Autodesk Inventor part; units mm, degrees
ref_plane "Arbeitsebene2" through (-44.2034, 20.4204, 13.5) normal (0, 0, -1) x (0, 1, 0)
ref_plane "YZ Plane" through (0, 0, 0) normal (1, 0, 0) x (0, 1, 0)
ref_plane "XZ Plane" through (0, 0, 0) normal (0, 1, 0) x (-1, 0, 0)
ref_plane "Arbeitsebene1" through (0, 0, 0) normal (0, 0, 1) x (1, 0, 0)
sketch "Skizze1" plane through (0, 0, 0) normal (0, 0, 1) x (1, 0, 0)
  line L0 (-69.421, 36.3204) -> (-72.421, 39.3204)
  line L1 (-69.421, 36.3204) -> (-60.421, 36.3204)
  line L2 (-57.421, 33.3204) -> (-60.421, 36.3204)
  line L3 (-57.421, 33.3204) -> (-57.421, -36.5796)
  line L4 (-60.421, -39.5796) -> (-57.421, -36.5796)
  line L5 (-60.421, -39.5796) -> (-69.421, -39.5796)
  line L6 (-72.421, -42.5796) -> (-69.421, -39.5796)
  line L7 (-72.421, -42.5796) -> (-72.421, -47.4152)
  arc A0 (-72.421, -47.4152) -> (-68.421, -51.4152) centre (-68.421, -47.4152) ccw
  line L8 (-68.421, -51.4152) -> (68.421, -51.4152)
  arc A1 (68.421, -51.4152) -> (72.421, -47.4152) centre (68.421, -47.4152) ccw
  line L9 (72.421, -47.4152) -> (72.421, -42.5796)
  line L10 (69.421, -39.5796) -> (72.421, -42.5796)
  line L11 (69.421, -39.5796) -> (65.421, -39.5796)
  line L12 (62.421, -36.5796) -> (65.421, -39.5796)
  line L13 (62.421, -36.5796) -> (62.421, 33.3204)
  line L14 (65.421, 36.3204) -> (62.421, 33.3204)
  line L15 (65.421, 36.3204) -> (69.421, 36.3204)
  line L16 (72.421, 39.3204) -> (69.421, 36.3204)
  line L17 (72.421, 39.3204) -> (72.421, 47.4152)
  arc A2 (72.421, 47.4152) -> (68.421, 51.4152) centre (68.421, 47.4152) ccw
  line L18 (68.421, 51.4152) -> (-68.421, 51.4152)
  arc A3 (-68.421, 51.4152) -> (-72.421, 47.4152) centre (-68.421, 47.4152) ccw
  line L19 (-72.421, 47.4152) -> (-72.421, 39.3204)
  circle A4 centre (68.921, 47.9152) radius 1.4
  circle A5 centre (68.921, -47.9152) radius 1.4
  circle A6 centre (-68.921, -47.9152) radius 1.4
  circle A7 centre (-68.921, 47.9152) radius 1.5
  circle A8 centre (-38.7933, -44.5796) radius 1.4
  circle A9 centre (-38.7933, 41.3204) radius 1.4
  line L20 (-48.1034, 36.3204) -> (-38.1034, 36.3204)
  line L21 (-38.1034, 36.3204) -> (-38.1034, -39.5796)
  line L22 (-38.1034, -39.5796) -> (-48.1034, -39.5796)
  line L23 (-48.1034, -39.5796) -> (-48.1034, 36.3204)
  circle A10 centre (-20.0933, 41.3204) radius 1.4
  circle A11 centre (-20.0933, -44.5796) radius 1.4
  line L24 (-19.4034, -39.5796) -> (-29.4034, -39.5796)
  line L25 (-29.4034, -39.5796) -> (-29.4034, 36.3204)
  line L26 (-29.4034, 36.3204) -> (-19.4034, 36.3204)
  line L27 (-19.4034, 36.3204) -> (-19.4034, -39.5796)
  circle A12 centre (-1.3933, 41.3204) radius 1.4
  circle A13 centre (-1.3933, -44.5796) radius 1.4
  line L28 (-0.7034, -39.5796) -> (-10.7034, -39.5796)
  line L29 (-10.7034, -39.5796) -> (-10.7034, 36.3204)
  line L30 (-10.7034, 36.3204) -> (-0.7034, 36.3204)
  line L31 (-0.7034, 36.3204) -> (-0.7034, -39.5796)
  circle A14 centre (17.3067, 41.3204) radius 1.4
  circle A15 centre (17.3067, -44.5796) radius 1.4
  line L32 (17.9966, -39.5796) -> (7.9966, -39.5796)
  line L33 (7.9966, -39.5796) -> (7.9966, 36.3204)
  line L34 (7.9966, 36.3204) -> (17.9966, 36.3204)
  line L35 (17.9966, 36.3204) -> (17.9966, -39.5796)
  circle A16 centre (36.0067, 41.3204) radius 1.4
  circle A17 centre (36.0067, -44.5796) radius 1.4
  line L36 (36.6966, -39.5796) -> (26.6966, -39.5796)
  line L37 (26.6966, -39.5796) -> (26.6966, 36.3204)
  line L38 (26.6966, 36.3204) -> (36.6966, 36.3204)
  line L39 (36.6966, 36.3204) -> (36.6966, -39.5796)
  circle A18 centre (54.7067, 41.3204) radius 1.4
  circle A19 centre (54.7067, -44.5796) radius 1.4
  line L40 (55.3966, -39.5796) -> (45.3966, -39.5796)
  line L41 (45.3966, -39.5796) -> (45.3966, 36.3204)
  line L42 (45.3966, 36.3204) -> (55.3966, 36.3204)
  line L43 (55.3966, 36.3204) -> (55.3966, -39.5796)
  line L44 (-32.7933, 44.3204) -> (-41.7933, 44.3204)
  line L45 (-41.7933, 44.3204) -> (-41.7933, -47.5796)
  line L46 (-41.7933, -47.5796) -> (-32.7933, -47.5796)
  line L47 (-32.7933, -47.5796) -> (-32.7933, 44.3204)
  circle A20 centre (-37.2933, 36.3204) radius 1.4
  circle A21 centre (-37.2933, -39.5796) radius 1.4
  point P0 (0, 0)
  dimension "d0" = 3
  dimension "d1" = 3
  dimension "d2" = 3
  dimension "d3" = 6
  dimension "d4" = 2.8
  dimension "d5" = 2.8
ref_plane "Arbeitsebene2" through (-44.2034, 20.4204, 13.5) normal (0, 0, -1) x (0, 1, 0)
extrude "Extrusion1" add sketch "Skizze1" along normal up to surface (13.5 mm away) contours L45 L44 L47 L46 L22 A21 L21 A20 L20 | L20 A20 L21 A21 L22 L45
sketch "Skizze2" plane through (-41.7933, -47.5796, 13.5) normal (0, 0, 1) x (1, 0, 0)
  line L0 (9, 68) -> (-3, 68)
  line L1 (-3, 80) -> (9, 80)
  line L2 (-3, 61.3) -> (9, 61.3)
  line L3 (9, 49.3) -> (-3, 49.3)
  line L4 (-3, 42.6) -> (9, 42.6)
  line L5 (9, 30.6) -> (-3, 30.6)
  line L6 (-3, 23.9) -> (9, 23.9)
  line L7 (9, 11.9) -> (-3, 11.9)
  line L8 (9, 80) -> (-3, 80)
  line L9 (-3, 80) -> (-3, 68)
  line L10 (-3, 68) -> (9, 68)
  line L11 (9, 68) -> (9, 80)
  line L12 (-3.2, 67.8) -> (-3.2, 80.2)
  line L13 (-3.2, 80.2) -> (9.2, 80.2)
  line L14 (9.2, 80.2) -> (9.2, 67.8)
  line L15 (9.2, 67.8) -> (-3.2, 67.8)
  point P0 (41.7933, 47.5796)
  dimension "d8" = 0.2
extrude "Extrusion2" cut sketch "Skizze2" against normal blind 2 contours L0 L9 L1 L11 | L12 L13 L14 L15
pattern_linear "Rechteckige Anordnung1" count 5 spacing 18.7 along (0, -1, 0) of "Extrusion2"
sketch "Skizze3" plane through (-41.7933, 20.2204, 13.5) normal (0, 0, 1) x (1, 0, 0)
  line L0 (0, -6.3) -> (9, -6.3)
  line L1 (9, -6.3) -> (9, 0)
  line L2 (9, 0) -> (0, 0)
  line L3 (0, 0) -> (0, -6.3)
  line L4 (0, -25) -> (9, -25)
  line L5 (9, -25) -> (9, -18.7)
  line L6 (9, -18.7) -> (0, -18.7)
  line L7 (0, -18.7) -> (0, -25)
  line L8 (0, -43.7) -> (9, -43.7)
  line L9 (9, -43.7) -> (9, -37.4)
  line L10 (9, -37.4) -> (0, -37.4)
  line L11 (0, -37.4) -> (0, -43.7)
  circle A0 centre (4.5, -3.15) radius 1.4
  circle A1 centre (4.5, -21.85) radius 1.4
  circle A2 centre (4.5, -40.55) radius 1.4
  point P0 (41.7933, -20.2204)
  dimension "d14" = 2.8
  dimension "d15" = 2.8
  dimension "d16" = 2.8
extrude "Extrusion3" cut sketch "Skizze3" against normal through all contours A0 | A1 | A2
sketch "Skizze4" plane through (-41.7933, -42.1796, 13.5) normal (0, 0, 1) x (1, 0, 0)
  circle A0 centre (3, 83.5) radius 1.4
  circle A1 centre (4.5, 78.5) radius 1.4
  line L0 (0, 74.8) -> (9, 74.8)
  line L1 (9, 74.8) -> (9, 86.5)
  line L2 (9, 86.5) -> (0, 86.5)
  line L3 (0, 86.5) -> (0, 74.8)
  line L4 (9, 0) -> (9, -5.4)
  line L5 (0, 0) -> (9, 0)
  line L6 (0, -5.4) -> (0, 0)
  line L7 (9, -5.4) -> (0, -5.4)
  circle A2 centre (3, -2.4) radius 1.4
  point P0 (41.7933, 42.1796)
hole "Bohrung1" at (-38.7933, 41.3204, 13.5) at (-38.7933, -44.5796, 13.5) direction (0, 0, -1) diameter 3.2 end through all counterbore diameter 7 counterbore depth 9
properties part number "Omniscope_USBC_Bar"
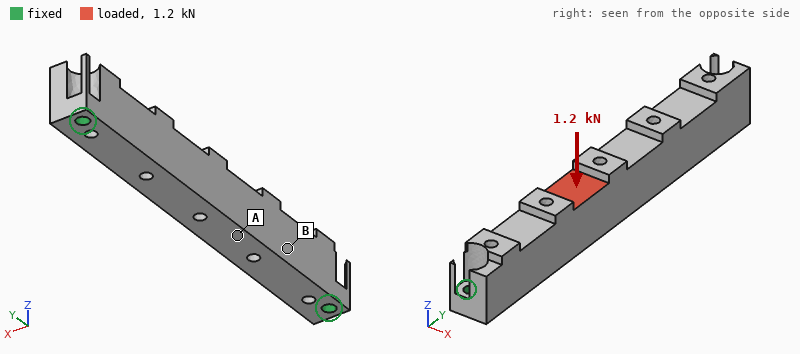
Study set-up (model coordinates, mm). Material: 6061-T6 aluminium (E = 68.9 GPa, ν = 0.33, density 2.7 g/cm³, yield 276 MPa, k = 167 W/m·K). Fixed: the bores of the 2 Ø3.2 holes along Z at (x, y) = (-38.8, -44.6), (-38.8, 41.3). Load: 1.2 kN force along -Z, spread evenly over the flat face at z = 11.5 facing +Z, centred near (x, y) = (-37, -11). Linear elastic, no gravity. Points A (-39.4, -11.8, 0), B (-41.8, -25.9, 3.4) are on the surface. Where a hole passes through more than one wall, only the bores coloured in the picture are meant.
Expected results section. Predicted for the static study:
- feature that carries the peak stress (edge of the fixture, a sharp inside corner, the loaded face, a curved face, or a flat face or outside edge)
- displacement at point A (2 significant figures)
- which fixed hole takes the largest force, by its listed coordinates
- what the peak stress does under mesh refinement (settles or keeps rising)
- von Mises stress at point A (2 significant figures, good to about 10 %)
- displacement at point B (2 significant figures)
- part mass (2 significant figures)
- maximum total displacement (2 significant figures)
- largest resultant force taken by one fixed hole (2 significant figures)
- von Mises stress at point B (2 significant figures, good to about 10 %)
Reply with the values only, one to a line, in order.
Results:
edge of the fixture
0.095 mm
(-38.8, -44.6)
keeps rising
60 MPa
0.058 mm
25 g
0.11 mm
1.3 kN
18 MPa
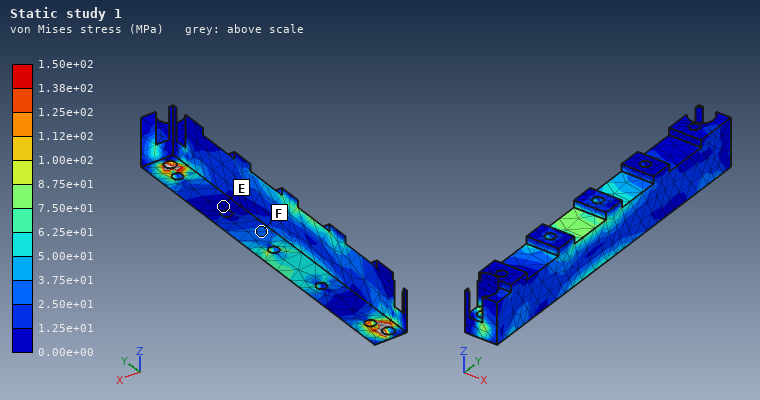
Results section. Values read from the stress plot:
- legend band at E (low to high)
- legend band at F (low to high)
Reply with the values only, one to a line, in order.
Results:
0.00e+00 to 1.25e+01 MPa
2.50e+01 to 3.75e+01 MPa
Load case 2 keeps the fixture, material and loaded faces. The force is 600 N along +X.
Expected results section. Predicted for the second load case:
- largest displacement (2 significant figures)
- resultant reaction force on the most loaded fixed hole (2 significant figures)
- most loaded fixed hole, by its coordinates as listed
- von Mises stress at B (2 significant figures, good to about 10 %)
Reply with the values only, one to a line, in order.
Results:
0.10 mm
400 N
(-38.8, -44.6)
16 MPa
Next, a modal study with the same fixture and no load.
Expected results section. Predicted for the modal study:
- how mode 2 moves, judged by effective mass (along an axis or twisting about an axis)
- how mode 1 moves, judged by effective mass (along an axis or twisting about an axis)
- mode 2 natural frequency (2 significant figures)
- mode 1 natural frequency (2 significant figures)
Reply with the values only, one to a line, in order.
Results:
along Z
along X
5100 Hz
4000 Hz
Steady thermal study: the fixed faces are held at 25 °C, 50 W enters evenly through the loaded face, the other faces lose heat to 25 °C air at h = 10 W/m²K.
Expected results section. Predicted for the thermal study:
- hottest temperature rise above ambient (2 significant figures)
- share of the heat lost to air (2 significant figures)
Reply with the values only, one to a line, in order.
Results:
76 K
3.4 %
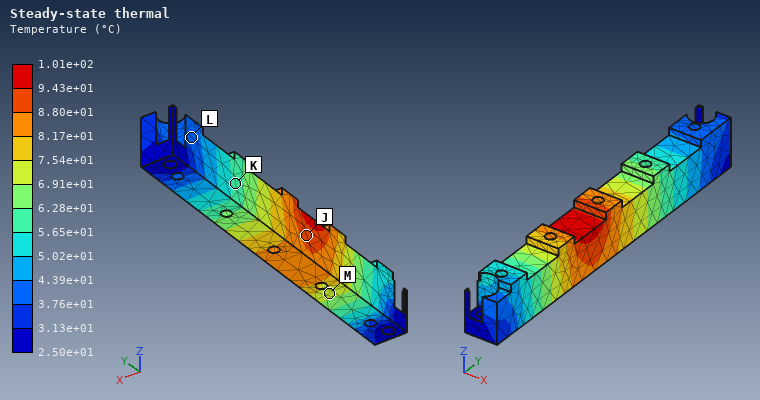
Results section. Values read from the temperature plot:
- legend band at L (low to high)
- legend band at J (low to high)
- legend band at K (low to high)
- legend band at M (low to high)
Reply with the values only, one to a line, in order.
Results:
3.76e+01 to 4.39e+01 °C
8.80e+01 to 9.43e+01 °C
5.65e+01 to 6.28e+01 °C
6.91e+01 to 7.54e+01 °C
